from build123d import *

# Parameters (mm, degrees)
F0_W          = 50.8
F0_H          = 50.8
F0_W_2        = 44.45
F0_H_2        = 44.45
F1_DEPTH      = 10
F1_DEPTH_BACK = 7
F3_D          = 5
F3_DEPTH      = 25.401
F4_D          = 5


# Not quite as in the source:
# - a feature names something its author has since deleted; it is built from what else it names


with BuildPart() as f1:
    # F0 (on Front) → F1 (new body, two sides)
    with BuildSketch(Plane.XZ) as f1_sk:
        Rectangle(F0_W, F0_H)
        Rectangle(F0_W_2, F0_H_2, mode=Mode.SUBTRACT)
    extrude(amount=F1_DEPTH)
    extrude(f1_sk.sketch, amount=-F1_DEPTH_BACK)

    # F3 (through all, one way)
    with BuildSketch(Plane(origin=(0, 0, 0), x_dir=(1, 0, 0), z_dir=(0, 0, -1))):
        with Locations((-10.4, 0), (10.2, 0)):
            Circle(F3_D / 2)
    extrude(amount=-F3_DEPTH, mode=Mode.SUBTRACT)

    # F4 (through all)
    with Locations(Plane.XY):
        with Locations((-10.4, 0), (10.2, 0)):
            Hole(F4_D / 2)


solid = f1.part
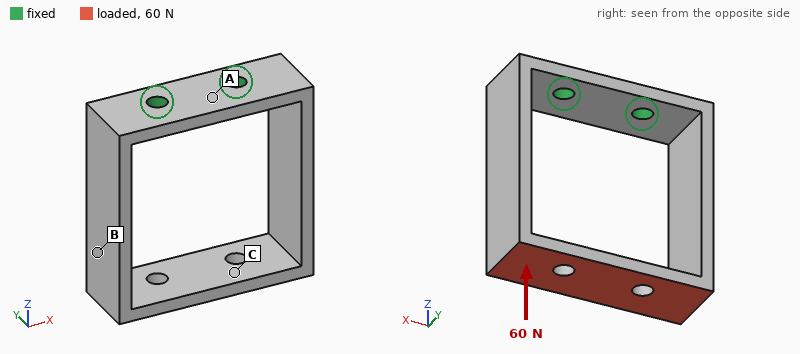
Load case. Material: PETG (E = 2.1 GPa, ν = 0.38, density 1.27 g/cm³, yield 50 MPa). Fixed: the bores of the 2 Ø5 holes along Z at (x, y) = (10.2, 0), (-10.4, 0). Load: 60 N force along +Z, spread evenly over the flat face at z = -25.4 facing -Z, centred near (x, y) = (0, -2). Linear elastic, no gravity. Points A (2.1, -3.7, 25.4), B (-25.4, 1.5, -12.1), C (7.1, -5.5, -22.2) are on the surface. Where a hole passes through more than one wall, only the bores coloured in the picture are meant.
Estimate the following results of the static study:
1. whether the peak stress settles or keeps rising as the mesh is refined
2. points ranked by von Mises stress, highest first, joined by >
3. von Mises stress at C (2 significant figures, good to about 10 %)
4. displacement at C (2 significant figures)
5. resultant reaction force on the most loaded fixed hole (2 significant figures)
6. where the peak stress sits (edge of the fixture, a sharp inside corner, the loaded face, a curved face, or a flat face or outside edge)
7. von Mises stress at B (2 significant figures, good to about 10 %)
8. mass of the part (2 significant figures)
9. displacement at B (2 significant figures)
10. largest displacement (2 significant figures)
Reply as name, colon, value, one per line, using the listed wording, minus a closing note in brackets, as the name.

whether the peak stress settles or keeps rising as the mesh is refined: keeps rising
points ranked by von Mises stress, highest first, joined by >: C > B > A
von Mises stress at C: 6.6 MPa
displacement at C: 0.60 mm
resultant reaction force on the most loaded fixed hole: 30 N
where the peak stress sits: edge of the fixture
von Mises stress at B: 3.3 MPa
mass of the part: 13 g
displacement at B: 0.26 mm
largest displacement: 0.68 mm
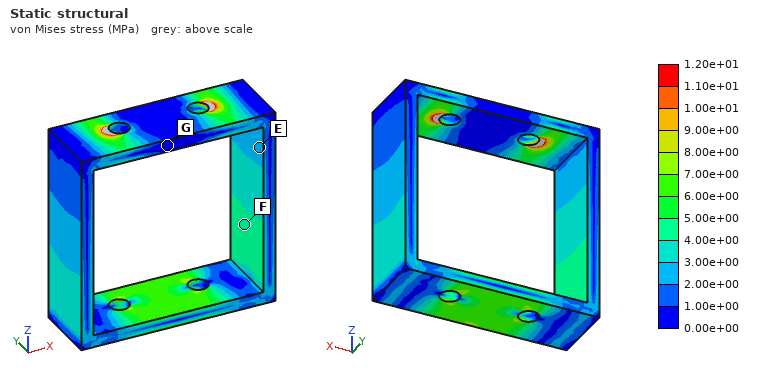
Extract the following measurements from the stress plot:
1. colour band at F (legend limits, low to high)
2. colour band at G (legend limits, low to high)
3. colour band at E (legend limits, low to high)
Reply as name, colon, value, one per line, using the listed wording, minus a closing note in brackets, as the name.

colour band at F: 4.00e+00 to 5.00e+00 MPa
colour band at G: 0.00e+00 to 1.00e+00 MPa
colour band at E: 2.00e+00 to 3.00e+00 MPa
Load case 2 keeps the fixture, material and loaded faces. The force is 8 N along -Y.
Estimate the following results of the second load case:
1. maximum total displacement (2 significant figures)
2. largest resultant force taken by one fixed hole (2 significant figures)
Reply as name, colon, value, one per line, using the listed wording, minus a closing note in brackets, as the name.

maximum total displacement: 0.78 mm
largest resultant force taken by one fixed hole: 4.4 N
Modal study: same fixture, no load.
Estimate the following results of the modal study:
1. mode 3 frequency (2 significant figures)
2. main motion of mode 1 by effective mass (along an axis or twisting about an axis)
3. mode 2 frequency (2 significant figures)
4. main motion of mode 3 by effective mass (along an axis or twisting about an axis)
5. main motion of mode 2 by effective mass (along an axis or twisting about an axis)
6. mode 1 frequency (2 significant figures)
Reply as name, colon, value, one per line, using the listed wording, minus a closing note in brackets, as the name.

mode 3 frequency: 450 Hz
main motion of mode 1 by effective mass: along X
mode 2 frequency: 230 Hz
main motion of mode 3 by effective mass: twisting about Z
main motion of mode 2 by effective mass: along Y
mode 1 frequency: 200 Hz
